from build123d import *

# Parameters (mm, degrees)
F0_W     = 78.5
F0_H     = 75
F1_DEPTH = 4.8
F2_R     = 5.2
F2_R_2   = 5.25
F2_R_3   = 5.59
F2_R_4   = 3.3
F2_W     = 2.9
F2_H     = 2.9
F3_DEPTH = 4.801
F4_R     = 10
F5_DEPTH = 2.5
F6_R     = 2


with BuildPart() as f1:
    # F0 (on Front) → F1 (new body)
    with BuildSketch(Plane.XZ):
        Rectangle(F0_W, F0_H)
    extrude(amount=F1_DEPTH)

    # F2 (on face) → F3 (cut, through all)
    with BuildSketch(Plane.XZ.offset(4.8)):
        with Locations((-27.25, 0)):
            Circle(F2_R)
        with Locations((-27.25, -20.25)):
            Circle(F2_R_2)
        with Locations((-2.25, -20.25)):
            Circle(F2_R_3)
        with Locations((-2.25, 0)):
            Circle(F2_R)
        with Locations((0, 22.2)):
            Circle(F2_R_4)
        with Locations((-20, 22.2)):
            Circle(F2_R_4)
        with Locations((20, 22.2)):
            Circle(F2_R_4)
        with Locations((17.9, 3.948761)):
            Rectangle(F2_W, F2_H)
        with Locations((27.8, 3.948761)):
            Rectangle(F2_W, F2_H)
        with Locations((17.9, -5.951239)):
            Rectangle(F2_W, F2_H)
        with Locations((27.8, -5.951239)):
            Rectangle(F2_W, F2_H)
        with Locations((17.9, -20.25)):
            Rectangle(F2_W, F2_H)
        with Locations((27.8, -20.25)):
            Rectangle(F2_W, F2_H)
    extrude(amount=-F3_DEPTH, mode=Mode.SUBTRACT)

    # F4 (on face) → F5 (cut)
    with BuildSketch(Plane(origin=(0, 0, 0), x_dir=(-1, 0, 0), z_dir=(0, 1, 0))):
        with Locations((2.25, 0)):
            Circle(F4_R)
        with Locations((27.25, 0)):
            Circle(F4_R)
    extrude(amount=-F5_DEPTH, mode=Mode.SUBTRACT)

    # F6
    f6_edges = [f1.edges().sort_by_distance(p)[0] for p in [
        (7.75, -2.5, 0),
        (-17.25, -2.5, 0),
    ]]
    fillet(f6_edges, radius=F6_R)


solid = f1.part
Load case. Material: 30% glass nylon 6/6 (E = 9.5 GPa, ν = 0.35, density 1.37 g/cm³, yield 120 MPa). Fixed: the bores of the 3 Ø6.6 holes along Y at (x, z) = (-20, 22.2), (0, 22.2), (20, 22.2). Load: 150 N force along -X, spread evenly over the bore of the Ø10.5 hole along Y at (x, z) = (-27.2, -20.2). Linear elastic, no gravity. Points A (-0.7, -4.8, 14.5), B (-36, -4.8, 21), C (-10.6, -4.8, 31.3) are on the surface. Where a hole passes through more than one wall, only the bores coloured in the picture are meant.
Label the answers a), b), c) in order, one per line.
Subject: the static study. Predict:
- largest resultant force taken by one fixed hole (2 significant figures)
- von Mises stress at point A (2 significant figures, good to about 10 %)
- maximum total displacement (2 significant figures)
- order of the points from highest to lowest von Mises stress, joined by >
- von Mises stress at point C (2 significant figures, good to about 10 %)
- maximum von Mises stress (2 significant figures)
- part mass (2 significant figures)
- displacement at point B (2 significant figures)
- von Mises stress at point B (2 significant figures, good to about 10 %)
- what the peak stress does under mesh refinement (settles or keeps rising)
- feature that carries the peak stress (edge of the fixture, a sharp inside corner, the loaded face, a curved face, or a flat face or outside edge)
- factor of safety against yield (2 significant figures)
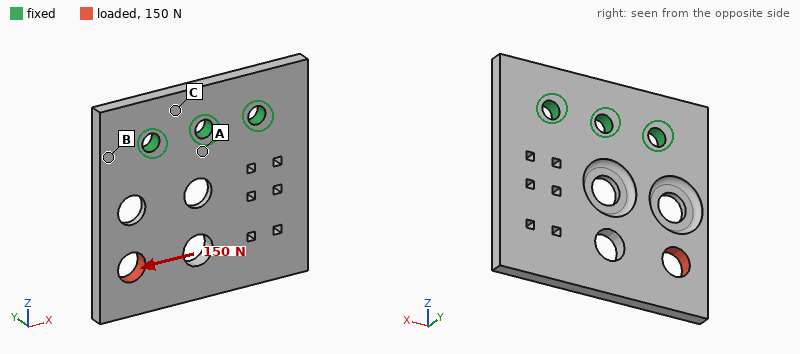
a) 150 N
b) 1.6 MPa
c) 25 µm
d) A > B > C
e) 0.42 MPa
f) 5.8 MPa
g) 34 g
h) 4.7 µm
i) 0.94 MPa
j) settles
k) a curved face
l) 21
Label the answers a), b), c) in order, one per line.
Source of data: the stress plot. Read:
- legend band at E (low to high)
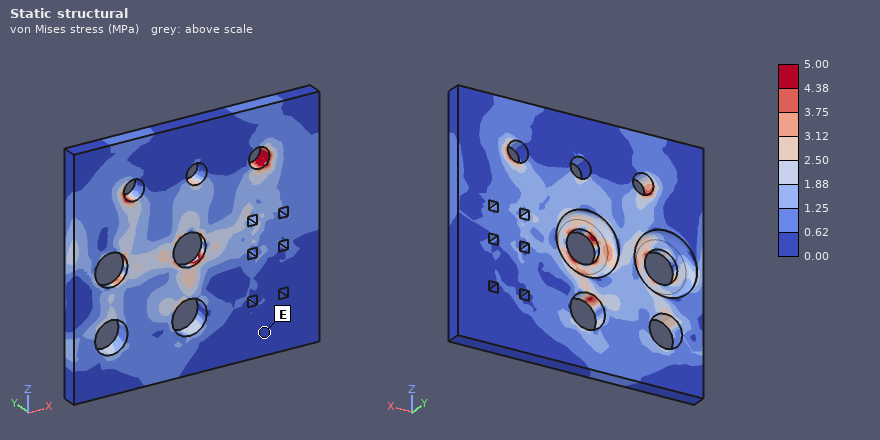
a) 0.00 to 0.62 MPa
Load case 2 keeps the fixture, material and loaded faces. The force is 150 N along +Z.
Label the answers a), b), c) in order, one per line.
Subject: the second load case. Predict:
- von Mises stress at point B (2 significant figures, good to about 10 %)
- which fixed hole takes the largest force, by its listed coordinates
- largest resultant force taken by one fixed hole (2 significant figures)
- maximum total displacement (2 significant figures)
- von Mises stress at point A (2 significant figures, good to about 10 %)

a) 0.91 MPa
b) (-20, 22.2)
c) 150 N
d) 34 µm
e) 0.44 MPa
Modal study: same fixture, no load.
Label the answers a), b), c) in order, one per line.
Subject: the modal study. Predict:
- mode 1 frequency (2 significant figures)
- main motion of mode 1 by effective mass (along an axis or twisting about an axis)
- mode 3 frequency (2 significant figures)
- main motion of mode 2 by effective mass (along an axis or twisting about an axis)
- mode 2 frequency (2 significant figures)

a) 540 Hz
b) along Y
c) 2400 Hz
d) twisting about Z
e) 1000 Hz
